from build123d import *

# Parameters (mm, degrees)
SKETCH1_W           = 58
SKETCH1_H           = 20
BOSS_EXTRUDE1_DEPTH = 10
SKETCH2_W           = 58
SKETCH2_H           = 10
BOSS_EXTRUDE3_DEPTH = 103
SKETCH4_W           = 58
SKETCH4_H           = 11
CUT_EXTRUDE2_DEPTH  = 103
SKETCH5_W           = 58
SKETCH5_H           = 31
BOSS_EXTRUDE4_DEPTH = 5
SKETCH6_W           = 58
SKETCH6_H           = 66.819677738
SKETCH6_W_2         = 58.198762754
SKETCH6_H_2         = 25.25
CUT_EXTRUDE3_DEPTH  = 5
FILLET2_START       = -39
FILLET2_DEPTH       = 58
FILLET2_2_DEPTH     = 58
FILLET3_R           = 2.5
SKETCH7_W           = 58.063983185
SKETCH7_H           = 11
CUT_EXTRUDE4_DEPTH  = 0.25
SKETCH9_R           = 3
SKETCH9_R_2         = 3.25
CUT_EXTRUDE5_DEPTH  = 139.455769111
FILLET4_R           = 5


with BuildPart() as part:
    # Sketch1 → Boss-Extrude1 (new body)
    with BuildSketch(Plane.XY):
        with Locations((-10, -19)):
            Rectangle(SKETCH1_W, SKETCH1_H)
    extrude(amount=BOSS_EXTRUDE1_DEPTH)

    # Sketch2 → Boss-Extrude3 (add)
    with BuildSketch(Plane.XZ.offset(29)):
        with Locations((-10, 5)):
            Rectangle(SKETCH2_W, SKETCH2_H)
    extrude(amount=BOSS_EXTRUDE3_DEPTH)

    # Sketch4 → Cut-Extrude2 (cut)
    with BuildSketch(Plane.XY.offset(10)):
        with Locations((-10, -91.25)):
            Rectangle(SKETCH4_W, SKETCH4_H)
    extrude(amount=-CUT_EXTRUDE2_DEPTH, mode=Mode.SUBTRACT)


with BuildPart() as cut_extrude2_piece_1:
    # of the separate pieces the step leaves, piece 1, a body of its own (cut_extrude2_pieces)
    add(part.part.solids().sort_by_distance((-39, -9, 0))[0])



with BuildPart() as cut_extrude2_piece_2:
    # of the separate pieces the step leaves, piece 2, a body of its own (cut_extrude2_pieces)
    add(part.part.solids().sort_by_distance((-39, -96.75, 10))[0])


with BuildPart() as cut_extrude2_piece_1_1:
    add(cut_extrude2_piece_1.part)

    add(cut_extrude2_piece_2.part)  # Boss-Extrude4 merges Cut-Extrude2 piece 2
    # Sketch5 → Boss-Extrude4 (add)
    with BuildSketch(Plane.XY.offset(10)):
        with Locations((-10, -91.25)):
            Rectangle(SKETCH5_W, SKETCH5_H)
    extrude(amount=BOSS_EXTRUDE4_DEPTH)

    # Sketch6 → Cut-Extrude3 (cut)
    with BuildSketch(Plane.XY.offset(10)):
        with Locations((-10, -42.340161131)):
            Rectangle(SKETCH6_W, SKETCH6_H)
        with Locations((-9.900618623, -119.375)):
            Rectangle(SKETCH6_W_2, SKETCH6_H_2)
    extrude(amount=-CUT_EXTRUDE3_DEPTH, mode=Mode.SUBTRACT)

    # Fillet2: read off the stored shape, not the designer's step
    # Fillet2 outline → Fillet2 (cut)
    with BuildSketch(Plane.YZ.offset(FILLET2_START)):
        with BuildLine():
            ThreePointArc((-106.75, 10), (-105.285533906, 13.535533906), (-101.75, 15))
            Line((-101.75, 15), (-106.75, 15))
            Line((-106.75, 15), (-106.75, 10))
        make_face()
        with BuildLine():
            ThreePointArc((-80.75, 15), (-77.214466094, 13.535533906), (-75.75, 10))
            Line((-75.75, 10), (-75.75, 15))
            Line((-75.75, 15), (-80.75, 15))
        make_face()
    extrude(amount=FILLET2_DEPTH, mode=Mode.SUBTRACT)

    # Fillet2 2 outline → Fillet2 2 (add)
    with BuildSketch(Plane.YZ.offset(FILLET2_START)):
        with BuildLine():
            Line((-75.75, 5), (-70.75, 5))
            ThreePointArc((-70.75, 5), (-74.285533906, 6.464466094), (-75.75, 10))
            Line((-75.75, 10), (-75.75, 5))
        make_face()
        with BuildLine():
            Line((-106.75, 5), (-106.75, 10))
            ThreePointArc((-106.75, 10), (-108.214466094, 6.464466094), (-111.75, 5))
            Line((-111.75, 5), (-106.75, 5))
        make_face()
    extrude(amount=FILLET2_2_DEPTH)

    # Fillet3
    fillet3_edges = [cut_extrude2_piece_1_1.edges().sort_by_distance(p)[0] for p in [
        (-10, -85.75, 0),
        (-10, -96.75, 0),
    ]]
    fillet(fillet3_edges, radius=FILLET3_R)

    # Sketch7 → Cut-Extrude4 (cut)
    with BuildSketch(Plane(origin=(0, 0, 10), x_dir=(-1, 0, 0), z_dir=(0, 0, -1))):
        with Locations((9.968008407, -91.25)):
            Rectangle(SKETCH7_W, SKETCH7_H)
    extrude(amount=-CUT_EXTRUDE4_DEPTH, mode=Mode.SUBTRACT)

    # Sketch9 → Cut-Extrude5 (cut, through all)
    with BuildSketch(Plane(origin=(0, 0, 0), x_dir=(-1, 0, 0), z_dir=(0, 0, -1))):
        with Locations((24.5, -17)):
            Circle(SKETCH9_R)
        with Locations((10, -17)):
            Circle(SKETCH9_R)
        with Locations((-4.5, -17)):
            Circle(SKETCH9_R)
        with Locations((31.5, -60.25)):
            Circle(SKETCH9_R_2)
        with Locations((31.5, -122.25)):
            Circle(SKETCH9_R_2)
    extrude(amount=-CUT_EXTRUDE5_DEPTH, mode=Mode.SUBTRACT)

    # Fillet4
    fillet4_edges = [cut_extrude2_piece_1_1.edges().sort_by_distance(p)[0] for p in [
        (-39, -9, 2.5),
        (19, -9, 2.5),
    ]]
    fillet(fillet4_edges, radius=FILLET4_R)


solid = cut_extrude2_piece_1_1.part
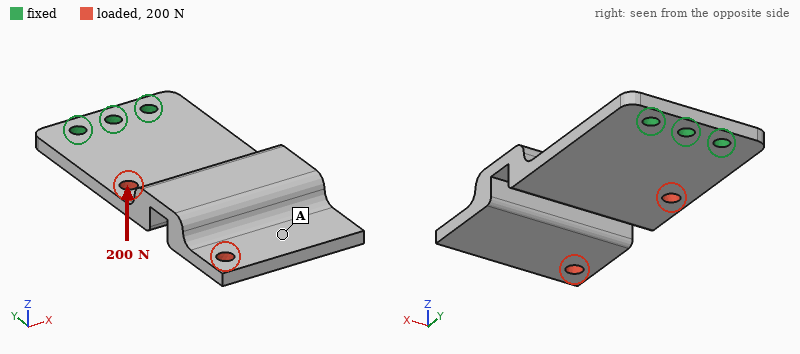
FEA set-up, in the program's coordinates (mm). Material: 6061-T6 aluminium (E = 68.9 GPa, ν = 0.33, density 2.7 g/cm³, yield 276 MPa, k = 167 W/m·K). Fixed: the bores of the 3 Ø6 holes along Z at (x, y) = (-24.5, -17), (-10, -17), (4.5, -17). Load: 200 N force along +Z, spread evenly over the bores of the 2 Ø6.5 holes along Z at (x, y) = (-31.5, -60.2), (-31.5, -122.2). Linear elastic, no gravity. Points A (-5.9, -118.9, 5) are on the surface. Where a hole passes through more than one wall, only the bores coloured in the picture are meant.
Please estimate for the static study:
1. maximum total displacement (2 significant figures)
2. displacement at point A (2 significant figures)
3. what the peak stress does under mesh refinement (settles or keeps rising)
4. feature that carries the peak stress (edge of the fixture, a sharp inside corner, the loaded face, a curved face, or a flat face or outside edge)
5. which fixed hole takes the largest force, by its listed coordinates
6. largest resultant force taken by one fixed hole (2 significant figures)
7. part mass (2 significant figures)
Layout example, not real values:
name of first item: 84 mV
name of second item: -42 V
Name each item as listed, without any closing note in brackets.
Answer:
maximum total displacement: 1.2 mm
displacement at point A: 0.96 mm
what the peak stress does under mesh refinement: keeps rising
feature that carries the peak stress: edge of the fixture
which fixed hole takes the largest force, by its listed coordinates: (-24.5, -17)
largest resultant force taken by one fixed hole: 150 N
part mass: 120 g
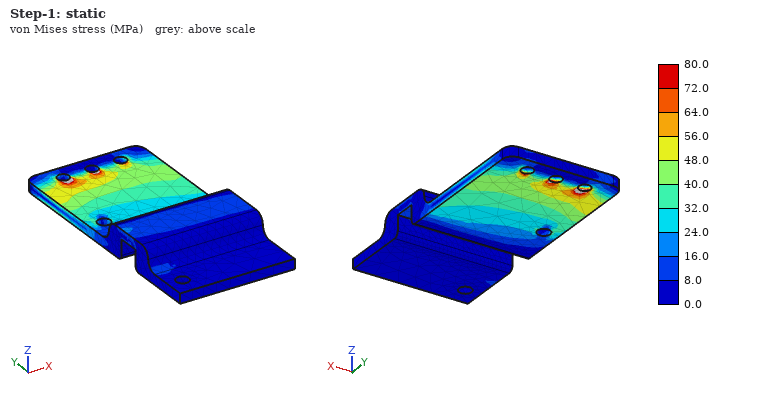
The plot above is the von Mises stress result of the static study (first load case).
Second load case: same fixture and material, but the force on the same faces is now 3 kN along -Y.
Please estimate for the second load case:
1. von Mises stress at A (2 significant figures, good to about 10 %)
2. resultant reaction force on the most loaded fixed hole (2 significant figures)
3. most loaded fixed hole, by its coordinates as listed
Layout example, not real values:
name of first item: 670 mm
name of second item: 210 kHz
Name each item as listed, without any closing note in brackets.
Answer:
von Mises stress at A: 8.1 MPa
resultant reaction force on the most loaded fixed hole: 3.0 kN
most loaded fixed hole, by its coordinates as listed: (-24.5, -17)
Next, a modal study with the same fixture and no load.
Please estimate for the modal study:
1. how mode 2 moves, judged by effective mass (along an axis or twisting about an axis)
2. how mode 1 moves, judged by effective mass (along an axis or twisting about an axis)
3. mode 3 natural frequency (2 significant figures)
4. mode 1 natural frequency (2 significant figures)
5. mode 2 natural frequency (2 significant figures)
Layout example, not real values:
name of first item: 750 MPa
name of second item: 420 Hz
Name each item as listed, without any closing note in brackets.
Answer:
how mode 2 moves, judged by effective mass: twisting about Y
how mode 1 moves, judged by effective mass: along Z
mode 3 natural frequency: 1900 Hz
mode 1 natural frequency: 280 Hz
mode 2 natural frequency: 1200 Hz
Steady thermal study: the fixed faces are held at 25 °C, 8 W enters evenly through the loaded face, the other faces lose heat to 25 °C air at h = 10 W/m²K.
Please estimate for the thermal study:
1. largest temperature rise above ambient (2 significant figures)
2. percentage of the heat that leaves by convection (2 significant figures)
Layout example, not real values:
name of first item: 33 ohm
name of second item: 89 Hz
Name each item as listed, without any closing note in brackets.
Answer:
largest temperature rise above ambient: 13 K
percentage of the heat that leaves by convection: 14 %
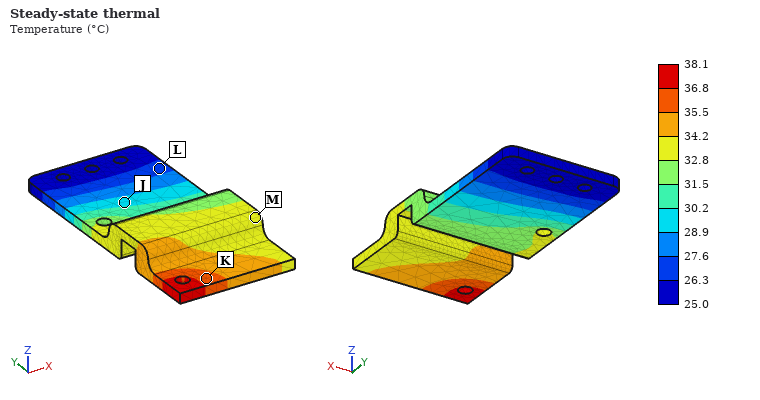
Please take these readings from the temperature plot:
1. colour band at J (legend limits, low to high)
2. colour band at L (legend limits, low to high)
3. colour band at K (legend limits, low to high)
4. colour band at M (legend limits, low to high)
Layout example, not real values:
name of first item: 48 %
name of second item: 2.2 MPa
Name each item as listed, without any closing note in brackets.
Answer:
colour band at J: 28.9 to 30.2 °C
colour band at L: 26.3 to 27.6 °C
colour band at K: 35.5 to 36.8 °C
colour band at M: 32.8 to 34.2 °C
